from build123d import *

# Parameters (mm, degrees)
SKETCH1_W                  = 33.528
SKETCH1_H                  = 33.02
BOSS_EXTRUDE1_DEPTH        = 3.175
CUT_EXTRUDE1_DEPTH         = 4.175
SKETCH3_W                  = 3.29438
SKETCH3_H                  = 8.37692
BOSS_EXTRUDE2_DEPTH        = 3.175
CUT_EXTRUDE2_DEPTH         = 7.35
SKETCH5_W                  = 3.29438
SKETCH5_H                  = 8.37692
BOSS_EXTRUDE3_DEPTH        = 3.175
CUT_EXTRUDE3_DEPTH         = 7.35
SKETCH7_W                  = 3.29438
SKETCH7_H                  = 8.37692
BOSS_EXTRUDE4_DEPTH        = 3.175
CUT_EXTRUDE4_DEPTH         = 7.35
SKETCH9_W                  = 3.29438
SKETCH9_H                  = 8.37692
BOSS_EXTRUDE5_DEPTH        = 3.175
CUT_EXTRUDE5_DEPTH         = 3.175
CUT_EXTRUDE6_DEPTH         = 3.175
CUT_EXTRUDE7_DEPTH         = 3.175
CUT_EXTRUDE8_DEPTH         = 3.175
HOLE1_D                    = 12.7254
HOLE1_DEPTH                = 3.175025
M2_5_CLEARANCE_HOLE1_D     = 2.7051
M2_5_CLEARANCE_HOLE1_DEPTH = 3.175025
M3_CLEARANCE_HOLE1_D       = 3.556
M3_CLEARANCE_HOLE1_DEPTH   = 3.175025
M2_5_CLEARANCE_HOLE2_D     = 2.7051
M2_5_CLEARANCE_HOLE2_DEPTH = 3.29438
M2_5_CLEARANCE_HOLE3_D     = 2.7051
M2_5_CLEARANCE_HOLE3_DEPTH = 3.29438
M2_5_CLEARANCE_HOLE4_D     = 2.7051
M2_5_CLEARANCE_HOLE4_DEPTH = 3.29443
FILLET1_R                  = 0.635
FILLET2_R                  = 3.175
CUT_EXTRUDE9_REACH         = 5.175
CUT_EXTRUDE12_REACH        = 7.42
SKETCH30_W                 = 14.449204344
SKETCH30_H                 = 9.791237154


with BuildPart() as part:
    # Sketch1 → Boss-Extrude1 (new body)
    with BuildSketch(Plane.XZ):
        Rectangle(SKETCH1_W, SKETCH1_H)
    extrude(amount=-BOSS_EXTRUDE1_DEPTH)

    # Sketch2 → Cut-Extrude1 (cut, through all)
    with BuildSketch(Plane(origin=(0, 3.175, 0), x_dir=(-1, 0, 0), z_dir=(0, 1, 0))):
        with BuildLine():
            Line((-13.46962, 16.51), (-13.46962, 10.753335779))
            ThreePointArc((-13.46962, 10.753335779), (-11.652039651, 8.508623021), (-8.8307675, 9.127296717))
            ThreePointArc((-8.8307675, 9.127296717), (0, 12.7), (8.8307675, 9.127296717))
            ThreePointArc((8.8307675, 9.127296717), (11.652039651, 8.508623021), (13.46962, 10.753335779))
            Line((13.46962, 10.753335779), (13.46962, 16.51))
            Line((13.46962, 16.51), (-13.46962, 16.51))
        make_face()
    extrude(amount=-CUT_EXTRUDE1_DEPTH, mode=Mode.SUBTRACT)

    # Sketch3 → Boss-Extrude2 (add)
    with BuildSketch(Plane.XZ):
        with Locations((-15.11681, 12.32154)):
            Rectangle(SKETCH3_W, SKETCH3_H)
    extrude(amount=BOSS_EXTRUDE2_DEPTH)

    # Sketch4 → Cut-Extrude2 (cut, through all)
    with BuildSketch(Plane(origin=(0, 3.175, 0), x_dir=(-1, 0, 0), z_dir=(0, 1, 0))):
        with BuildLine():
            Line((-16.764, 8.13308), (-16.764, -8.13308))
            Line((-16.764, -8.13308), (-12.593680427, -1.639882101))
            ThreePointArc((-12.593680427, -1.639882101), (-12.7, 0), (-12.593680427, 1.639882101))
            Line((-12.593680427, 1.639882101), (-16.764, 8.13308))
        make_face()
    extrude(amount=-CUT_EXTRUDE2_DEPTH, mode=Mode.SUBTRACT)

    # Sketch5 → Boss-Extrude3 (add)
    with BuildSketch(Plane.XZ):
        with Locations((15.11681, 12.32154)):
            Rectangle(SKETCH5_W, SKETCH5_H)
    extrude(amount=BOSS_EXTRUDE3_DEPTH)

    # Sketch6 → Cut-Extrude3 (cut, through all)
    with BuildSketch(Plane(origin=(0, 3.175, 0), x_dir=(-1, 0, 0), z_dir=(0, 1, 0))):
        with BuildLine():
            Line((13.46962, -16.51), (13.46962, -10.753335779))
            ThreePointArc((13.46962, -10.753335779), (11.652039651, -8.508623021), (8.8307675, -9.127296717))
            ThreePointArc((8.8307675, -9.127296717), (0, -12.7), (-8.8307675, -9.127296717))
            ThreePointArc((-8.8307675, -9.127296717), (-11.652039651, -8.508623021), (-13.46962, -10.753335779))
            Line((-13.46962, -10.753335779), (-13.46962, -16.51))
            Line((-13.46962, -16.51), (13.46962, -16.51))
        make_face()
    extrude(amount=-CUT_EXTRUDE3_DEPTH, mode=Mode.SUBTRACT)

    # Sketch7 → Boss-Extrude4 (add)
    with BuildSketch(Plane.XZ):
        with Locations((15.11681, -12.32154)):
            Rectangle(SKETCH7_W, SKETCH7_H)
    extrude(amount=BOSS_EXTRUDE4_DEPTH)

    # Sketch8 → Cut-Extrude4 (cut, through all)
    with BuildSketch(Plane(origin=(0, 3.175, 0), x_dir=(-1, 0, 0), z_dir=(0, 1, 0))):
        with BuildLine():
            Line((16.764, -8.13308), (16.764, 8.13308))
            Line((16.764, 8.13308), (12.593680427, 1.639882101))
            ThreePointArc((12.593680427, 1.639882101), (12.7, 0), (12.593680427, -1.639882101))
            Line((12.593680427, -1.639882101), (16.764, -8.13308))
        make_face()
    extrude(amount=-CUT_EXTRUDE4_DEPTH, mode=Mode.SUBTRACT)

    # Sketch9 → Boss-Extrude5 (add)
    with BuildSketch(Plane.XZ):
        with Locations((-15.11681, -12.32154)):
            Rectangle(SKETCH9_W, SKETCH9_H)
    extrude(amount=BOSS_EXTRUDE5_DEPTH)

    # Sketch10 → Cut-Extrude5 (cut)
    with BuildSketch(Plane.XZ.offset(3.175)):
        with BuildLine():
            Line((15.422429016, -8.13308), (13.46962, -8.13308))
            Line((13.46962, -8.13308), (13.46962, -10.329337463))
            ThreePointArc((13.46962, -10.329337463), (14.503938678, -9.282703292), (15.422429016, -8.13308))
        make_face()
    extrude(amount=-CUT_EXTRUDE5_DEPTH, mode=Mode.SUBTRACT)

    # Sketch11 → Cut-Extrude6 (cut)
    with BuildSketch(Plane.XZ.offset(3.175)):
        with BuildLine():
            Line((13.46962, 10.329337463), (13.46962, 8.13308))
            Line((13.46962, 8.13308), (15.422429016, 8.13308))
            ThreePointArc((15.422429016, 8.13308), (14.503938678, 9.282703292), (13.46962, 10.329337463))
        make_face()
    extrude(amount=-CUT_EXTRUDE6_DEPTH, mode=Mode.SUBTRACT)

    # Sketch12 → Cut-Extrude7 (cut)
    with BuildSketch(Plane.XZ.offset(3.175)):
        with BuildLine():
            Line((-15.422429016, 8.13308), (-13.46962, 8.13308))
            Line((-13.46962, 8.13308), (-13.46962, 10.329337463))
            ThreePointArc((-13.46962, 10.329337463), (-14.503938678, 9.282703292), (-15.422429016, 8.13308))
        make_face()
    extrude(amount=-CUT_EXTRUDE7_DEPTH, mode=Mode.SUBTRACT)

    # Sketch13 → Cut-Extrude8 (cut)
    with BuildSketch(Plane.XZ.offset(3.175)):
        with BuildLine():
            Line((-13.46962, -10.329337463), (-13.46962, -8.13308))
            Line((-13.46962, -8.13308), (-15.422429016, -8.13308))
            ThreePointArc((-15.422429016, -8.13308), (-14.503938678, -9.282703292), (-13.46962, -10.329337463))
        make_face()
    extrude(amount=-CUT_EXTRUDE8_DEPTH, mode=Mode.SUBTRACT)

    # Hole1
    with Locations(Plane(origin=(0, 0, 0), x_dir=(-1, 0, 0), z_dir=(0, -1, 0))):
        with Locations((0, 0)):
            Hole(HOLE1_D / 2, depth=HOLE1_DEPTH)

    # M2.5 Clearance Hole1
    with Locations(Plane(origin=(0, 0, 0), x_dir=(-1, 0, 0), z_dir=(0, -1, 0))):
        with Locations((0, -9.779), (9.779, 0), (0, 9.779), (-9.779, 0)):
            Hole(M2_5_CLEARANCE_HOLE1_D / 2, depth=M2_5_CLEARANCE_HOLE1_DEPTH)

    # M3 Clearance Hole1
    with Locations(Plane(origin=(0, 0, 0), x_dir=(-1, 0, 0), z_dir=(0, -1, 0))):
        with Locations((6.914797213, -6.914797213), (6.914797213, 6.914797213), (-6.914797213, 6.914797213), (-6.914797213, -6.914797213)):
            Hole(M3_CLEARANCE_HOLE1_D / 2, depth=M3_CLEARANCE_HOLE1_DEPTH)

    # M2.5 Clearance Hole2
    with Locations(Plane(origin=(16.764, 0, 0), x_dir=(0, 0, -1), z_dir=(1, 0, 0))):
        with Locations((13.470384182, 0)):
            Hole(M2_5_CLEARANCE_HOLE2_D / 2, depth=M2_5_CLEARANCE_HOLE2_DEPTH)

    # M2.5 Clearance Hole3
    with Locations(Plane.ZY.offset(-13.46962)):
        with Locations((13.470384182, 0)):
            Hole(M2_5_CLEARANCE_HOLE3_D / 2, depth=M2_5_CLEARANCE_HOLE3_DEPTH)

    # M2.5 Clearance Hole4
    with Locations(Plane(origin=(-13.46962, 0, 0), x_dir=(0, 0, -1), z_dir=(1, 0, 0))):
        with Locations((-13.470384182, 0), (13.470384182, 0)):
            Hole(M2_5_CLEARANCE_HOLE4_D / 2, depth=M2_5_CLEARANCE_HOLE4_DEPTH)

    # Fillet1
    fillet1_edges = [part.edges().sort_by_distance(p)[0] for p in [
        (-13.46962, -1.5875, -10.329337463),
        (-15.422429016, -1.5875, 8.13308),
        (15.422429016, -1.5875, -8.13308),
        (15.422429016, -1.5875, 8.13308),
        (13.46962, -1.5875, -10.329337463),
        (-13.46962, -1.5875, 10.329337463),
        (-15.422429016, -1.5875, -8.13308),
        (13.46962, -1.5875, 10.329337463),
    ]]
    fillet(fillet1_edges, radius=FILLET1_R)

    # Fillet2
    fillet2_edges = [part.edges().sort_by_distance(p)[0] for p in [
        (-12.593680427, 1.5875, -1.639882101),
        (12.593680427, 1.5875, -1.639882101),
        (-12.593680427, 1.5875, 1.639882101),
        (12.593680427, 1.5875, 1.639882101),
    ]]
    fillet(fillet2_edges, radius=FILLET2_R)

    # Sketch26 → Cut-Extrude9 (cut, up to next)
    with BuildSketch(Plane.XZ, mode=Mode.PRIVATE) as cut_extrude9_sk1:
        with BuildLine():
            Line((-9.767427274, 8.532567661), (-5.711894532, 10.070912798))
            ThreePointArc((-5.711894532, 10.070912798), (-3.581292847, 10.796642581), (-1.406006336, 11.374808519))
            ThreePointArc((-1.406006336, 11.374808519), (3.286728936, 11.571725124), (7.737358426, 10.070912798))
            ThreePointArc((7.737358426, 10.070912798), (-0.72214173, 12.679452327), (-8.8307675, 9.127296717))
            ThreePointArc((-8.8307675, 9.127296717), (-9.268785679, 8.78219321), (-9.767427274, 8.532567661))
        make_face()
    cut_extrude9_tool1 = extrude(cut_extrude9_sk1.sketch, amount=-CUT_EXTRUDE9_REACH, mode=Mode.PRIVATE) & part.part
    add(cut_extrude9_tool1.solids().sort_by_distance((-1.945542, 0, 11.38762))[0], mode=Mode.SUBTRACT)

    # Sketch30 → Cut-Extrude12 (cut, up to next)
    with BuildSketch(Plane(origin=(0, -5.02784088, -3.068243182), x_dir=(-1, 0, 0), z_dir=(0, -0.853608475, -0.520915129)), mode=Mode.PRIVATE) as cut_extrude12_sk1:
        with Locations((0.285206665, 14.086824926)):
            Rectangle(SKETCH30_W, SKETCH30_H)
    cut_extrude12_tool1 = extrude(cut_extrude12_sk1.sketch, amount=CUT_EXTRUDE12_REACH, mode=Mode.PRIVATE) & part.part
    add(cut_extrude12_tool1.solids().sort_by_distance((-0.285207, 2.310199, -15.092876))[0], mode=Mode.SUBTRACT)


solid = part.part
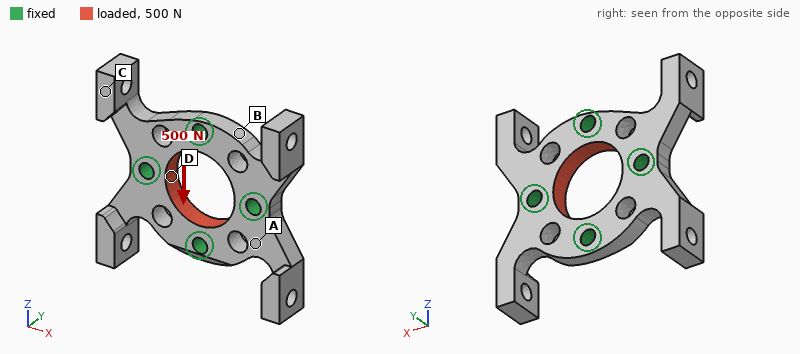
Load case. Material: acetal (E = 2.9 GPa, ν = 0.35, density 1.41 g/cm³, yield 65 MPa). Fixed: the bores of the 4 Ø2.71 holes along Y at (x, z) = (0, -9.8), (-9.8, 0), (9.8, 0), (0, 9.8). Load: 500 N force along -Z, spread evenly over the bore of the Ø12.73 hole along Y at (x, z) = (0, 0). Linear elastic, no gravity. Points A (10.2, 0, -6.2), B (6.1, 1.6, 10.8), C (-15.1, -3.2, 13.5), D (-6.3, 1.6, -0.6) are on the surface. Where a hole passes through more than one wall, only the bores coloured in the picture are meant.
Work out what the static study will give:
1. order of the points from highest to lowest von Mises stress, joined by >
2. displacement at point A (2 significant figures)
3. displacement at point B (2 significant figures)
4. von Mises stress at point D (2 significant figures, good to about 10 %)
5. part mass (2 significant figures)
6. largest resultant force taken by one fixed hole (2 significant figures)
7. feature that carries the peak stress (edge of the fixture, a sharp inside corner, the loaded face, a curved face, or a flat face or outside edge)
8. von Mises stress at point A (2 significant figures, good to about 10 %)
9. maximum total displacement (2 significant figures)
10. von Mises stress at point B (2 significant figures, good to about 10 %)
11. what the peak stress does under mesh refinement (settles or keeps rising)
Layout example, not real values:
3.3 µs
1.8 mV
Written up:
D > B > A > C
7.6 µm
9.7 µm
6.9 MPa
2.6 g
130 N
edge of the fixture
3.0 MPa
22 µm
4.9 MPa
keeps rising
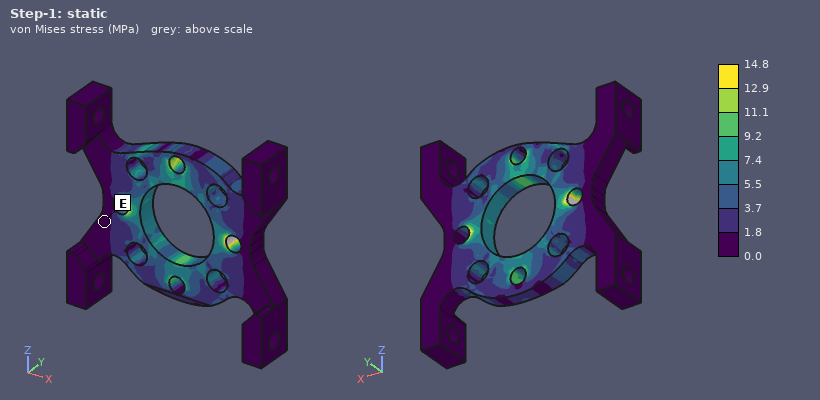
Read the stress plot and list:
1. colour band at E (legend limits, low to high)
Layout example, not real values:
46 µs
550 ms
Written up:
0.0 to 1.8 MPa
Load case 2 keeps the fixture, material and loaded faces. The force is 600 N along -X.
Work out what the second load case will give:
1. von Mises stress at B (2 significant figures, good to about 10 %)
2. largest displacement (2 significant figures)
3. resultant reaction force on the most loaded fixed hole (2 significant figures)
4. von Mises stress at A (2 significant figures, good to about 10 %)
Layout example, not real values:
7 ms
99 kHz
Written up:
6.6 MPa
27 µm
150 N
3.3 MPa
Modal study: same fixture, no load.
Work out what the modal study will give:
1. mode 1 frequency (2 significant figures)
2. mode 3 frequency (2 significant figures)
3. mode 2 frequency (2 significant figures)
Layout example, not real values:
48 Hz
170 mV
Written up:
2600 Hz
2600 Hz
2600 Hz
